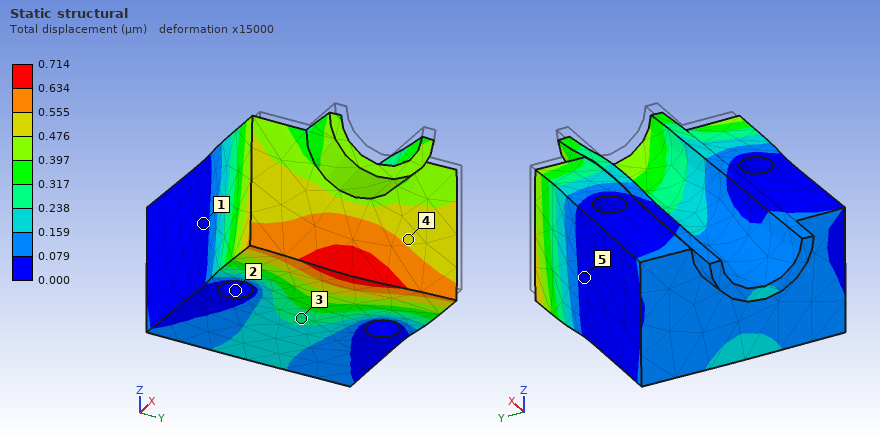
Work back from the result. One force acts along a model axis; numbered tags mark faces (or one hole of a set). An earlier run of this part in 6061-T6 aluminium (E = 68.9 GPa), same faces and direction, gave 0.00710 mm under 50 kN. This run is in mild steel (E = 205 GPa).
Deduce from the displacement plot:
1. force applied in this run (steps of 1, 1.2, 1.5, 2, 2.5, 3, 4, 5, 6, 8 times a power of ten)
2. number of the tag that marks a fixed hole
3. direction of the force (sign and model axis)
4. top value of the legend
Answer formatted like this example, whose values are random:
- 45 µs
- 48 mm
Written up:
- 15 kN
- 2
- -X
- 0.714 µm
